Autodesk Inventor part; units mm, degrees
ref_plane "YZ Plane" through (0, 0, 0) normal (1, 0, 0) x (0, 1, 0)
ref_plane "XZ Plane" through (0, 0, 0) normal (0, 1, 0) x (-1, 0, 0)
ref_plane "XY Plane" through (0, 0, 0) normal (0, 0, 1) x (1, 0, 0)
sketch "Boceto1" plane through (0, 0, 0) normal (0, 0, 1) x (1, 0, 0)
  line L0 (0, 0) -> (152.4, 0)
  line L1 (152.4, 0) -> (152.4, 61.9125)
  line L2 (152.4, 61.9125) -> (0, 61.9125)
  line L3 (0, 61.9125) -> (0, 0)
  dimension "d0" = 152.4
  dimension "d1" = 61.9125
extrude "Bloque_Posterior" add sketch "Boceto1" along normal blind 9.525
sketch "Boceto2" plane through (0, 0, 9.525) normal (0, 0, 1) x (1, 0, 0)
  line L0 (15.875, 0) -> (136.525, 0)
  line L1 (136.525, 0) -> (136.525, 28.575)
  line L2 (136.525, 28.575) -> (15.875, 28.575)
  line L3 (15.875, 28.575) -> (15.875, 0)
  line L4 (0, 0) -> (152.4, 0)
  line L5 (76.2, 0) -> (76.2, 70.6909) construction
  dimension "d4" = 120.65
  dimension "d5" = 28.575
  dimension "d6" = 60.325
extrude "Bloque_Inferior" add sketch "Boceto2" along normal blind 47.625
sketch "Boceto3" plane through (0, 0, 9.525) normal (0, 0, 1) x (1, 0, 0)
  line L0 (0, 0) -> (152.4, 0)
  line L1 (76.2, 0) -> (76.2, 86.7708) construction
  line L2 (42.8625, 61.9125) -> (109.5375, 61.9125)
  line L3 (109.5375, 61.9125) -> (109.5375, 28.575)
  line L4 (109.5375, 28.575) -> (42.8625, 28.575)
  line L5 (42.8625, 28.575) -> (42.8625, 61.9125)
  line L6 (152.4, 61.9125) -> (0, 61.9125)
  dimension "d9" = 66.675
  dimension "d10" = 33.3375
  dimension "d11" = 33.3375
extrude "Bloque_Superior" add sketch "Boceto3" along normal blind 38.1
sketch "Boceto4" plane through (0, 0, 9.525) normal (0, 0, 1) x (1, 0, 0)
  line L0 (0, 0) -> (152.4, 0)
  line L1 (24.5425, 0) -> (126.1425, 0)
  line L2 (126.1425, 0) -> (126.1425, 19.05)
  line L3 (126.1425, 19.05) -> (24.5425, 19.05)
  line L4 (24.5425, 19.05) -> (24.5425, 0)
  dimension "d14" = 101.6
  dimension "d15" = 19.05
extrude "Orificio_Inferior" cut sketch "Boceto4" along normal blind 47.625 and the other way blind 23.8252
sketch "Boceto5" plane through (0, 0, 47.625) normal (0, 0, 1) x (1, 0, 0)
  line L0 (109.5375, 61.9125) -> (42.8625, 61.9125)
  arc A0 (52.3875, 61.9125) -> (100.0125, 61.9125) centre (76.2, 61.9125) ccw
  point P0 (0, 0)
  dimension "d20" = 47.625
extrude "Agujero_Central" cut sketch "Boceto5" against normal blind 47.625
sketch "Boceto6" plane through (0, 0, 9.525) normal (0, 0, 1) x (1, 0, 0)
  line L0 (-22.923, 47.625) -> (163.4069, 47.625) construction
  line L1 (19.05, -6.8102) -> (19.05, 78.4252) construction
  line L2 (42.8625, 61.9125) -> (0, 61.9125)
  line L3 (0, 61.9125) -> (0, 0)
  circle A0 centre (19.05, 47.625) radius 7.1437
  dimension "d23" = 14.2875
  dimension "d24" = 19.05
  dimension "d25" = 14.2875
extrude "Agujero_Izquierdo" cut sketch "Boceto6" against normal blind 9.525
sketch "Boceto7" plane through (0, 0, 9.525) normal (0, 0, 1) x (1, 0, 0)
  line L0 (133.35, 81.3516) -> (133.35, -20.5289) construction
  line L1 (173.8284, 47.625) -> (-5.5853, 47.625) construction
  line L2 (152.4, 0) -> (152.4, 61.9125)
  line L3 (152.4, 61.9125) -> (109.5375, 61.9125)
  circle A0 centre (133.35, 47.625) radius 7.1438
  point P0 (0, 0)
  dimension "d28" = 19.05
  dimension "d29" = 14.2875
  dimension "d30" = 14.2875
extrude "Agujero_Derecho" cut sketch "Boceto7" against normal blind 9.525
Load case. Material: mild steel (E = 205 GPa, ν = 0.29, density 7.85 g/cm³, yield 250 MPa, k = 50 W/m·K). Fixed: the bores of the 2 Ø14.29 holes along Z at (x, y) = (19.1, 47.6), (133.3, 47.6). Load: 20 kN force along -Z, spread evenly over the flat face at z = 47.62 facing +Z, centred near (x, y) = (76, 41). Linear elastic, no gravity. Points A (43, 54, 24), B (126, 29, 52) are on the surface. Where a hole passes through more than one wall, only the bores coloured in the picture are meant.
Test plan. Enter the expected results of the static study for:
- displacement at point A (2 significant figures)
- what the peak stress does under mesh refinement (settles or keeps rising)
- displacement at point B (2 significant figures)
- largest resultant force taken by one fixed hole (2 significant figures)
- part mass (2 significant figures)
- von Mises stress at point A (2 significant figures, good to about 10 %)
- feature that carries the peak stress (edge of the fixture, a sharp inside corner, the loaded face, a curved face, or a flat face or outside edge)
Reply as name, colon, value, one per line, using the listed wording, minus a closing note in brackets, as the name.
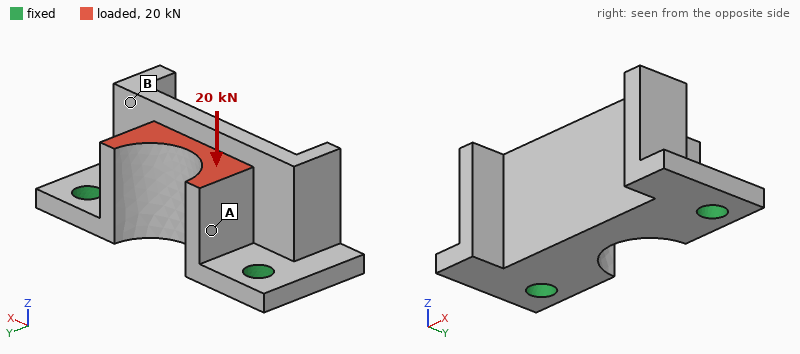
displacement at point A: 25 µm
what the peak stress does under mesh refinement: keeps rising
displacement at point B: 18 µm
largest resultant force taken by one fixed hole: 11 kN
part mass: 1.4 kg
von Mises stress at point A: 31 MPa
feature that carries the peak stress: edge of the fixture
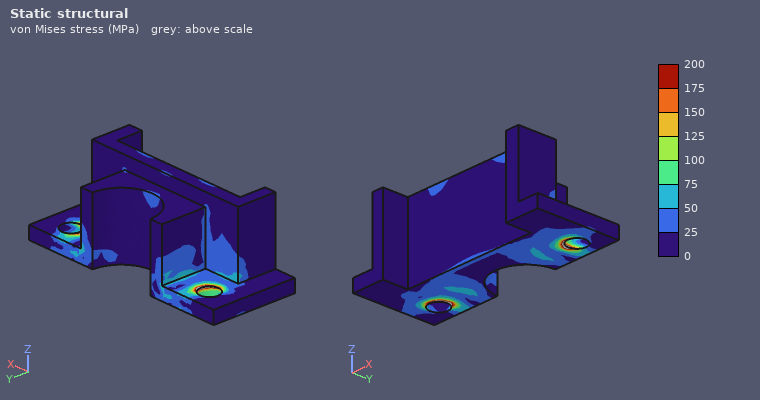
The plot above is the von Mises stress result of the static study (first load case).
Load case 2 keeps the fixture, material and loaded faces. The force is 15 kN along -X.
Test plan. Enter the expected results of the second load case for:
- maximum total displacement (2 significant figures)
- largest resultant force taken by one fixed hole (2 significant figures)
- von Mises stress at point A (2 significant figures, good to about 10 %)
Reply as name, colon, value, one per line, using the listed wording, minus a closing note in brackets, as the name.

maximum total displacement: 42 µm
largest resultant force taken by one fixed hole: 9.8 kN
von Mises stress at point A: 31 MPa
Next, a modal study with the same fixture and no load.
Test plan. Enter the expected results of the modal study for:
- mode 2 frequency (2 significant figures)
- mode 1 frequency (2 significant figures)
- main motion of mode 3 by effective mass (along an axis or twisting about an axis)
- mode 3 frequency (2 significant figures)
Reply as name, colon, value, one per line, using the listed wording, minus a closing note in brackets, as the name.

mode 2 frequency: 3500 Hz
mode 1 frequency: 1700 Hz
main motion of mode 3 by effective mass: along Z
mode 3 frequency: 4800 Hz
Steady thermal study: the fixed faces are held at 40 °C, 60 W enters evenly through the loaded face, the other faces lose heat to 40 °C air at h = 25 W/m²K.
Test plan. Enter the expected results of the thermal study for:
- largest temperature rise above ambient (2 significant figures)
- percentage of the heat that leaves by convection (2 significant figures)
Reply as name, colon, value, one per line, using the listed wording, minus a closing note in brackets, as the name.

largest temperature rise above ambient: 47 K
percentage of the heat that leaves by convection: 31 %
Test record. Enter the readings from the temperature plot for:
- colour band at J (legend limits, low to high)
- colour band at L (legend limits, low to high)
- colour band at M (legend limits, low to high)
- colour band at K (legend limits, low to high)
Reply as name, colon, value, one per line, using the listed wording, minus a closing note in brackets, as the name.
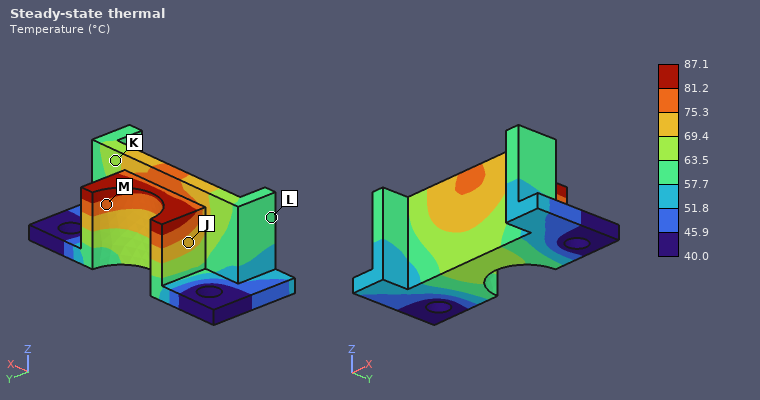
colour band at J: 69.4 to 75.3 °C
colour band at L: 57.7 to 63.5 °C
colour band at M: 75.3 to 81.2 °C
colour band at K: 63.5 to 69.4 °C
